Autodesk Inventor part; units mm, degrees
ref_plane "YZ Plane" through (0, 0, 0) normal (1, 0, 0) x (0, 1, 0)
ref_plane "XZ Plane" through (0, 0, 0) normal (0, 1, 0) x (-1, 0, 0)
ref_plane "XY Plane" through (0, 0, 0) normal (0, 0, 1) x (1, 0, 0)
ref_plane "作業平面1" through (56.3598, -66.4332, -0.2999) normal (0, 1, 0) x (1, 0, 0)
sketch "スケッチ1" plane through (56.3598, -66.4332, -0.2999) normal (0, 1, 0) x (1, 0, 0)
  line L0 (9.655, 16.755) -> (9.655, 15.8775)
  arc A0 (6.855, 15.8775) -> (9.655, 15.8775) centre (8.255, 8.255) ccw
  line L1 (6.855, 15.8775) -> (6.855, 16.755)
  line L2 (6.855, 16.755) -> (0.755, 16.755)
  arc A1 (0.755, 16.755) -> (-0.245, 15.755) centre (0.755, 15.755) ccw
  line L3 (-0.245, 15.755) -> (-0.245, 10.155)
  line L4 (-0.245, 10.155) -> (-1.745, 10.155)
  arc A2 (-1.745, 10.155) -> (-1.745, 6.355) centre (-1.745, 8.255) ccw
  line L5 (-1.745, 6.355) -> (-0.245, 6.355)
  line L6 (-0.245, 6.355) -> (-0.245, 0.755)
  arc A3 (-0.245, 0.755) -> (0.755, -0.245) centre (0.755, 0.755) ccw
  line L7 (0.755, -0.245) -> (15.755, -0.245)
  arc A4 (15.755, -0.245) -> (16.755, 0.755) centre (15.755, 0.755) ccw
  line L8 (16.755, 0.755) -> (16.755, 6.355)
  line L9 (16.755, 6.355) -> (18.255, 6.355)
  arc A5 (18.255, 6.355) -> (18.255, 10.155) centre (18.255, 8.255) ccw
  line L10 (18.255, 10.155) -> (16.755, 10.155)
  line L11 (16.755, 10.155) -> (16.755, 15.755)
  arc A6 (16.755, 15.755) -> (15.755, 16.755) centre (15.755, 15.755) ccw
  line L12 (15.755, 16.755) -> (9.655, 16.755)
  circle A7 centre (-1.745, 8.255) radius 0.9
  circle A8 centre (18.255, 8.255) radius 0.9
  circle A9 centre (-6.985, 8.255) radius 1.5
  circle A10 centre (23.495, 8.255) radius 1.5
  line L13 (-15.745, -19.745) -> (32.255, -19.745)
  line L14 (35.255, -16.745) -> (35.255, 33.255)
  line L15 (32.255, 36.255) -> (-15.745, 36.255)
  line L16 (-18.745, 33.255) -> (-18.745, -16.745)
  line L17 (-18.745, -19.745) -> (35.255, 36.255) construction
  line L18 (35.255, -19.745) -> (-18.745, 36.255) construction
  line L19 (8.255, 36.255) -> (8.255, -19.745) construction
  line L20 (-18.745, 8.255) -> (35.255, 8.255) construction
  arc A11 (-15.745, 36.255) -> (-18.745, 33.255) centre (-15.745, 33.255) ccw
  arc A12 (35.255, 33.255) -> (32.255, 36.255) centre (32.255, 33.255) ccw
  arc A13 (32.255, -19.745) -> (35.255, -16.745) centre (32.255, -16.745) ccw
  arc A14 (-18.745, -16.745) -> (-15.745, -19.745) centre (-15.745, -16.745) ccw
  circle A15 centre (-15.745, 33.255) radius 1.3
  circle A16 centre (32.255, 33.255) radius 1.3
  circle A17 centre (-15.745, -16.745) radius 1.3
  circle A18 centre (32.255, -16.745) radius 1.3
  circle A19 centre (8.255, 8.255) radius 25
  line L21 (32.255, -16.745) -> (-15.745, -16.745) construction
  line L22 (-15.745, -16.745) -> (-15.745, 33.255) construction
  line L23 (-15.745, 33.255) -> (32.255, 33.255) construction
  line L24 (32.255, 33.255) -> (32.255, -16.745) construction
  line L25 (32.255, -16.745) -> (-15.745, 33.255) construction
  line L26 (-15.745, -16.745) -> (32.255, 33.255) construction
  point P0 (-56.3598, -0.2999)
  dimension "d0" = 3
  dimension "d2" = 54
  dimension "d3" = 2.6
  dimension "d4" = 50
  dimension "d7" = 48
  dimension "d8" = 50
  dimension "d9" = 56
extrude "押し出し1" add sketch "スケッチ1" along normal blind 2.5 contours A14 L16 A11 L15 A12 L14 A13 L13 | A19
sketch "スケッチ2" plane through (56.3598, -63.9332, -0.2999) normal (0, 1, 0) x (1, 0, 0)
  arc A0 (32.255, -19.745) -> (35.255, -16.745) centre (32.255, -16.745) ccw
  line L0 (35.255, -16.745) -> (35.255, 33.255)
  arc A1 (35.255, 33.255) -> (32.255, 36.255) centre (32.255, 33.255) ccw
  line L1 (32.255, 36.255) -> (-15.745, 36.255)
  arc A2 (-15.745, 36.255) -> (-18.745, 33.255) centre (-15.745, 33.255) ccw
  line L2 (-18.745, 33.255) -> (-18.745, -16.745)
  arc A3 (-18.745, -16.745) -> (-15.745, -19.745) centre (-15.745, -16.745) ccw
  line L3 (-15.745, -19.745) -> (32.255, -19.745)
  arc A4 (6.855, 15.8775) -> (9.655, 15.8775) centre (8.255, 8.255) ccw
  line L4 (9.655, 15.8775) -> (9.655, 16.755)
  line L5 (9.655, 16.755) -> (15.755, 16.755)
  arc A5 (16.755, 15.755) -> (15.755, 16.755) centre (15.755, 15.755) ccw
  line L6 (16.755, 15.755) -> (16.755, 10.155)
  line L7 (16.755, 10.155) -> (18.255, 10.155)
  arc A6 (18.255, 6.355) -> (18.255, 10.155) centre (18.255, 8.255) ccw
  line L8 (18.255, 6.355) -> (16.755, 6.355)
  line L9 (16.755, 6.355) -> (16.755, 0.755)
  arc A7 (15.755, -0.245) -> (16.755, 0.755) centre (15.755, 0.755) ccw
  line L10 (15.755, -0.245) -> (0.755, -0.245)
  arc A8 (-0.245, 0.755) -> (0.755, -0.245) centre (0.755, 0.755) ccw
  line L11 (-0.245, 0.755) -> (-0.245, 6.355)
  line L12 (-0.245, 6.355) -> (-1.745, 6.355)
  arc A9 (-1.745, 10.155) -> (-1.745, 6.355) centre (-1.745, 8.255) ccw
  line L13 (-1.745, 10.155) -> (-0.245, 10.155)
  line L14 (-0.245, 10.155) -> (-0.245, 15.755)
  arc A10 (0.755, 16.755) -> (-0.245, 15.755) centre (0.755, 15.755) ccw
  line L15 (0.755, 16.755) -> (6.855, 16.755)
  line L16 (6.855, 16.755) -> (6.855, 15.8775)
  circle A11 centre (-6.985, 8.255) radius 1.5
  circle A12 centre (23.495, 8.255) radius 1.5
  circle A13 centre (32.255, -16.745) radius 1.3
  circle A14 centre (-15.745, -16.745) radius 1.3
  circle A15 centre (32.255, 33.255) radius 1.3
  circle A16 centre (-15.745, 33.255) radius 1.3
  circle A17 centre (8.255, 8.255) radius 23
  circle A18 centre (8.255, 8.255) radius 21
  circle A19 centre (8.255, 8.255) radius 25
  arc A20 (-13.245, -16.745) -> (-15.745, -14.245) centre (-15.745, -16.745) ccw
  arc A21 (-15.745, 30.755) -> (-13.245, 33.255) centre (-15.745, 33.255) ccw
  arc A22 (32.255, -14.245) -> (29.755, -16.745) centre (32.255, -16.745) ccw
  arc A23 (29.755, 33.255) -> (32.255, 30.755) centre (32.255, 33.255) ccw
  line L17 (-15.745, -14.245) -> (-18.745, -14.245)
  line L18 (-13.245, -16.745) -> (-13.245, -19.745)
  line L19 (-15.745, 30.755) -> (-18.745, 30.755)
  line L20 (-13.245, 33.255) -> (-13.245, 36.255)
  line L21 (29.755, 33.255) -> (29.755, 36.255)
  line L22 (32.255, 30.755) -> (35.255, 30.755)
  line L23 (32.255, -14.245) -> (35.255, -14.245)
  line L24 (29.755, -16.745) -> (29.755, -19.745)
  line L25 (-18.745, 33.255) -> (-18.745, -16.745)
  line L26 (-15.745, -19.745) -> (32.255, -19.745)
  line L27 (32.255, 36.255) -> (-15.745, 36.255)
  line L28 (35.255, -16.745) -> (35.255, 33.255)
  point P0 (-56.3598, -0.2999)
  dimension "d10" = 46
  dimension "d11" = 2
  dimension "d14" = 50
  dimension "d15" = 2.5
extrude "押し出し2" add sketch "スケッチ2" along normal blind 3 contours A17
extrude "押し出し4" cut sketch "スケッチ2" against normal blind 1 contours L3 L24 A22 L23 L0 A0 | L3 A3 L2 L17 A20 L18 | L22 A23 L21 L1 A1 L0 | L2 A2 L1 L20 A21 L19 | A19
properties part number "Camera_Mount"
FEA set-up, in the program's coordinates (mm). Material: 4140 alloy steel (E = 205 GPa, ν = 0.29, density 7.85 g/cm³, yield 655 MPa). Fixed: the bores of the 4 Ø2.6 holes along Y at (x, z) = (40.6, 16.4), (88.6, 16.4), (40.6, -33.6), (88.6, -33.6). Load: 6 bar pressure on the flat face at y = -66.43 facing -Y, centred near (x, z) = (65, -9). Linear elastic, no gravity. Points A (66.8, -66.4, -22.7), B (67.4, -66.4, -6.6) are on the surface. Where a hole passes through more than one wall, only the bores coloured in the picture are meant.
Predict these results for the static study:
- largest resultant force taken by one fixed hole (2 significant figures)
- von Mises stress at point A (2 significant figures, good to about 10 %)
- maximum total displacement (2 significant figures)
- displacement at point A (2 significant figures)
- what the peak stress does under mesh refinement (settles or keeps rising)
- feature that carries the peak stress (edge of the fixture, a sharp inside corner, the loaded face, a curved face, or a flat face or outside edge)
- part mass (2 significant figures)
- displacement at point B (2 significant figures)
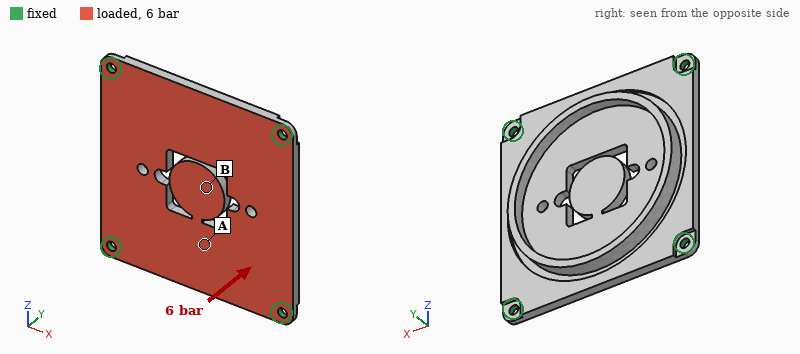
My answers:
730 N
95 MPa
0.31 mm
0.099 mm
keeps rising
edge of the fixture
60 g
0.24 mm
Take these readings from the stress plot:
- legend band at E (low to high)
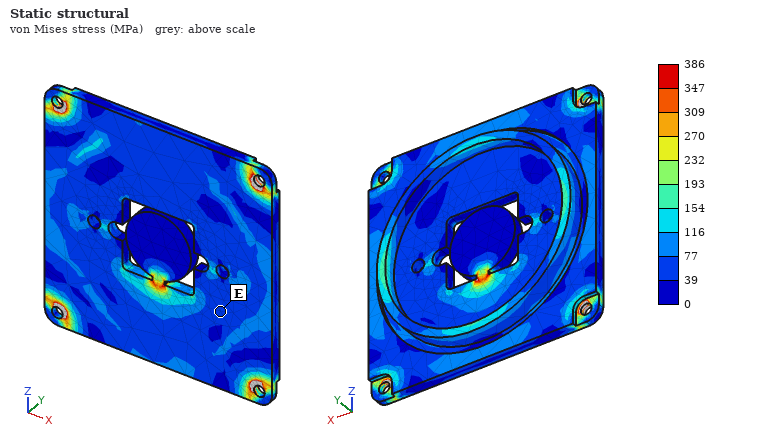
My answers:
39 to 77 MPa
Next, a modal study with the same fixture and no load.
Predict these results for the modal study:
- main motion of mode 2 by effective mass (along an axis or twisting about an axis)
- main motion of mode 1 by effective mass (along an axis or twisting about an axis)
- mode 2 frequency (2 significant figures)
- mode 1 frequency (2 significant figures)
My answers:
along Y
along Y
3800 Hz
2400 Hz
